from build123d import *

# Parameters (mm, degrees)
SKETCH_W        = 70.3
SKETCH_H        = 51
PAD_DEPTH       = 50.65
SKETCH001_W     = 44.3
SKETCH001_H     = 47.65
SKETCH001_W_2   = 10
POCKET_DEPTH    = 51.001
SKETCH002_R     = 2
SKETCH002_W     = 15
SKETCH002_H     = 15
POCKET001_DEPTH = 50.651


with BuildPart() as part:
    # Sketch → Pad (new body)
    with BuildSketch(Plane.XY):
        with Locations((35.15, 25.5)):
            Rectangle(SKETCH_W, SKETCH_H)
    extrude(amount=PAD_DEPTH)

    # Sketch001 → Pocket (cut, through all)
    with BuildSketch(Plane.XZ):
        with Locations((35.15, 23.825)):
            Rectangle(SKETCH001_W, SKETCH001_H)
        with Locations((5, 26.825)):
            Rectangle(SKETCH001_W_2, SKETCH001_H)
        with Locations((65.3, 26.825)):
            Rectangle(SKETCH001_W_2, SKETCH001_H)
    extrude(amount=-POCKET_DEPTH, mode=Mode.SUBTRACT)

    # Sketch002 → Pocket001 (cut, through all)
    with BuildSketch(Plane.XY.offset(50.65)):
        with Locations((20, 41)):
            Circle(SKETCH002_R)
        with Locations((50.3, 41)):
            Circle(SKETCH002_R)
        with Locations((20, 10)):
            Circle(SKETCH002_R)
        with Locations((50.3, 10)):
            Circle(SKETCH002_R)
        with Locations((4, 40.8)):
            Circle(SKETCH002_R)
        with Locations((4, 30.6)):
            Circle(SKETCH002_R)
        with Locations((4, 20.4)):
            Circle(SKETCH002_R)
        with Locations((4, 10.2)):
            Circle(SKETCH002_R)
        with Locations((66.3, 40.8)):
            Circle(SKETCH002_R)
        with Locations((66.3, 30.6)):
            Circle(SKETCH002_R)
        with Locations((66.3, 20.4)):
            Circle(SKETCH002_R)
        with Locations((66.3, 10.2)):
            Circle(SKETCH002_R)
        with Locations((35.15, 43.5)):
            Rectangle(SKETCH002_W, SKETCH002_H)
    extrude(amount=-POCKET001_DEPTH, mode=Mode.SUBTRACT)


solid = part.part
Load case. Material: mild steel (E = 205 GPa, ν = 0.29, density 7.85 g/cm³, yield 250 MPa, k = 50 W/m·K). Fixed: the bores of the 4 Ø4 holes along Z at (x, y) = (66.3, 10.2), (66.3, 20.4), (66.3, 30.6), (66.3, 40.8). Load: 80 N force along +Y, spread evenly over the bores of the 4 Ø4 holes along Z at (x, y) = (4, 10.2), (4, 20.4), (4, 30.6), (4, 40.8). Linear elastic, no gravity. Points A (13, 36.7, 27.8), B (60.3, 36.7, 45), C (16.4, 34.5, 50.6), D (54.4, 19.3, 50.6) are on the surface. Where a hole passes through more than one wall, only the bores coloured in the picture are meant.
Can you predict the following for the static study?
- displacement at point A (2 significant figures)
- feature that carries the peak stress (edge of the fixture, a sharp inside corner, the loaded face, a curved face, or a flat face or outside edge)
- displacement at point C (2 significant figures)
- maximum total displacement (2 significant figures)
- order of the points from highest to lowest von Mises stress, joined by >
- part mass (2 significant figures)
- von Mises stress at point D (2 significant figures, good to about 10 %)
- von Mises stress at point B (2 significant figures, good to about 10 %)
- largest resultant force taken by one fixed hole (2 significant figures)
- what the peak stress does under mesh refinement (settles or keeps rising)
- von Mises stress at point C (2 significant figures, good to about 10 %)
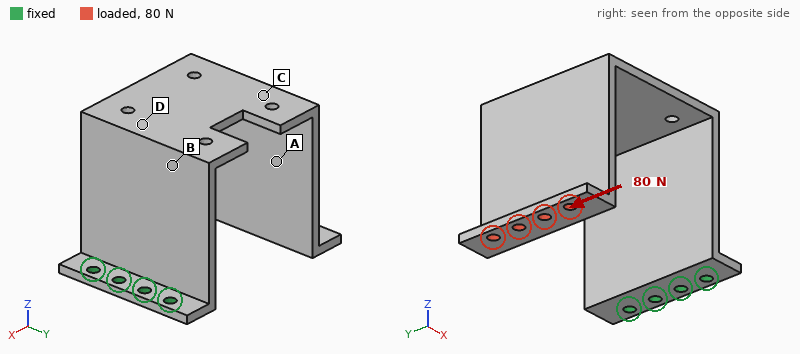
0.36 mm
a sharp inside corner
0.20 mm
0.61 mm
D > B > C > A
190 g
57 MPa
43 MPa
140 N
keeps rising
27 MPa
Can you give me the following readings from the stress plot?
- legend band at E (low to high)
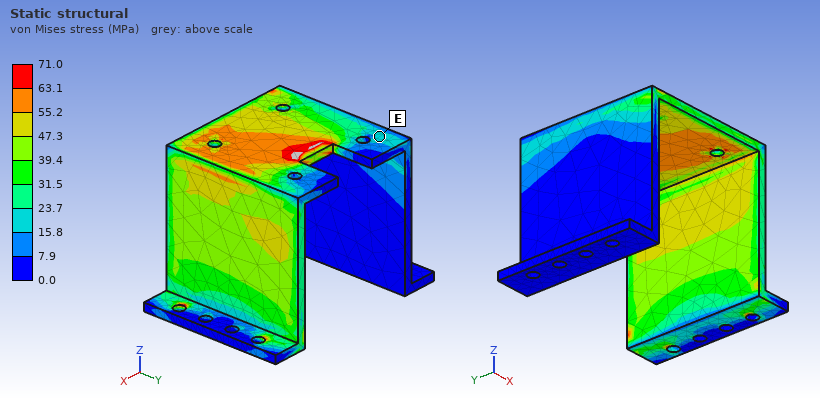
15.8 to 23.7 MPa
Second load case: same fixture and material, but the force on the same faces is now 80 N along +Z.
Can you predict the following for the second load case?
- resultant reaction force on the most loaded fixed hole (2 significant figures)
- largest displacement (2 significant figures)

41 N
1.0 mm
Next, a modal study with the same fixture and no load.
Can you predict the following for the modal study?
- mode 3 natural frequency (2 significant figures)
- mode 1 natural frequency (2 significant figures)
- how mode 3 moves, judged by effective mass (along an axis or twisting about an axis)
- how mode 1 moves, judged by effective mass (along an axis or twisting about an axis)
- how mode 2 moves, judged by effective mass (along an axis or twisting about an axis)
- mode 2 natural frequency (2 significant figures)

340 Hz
180 Hz
along X
along Z
along Y
280 Hz
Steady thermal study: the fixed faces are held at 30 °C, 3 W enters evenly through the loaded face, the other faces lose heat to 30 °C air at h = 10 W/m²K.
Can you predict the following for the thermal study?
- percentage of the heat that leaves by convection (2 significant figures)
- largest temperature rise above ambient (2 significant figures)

73 %
32 K
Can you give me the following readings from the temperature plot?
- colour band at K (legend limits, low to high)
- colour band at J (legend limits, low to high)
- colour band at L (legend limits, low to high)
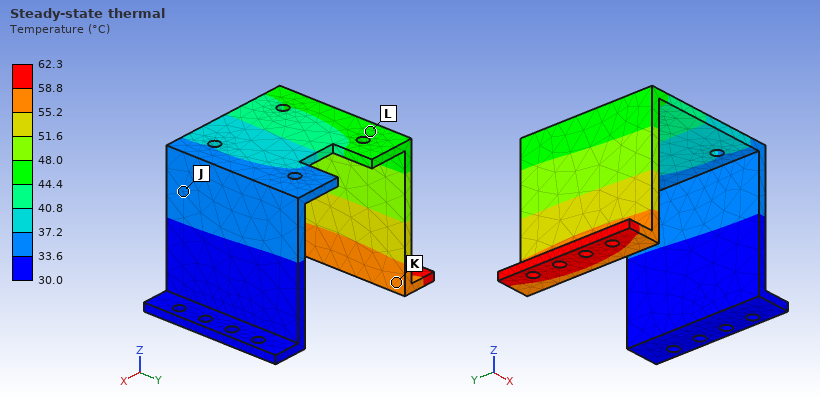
55.2 to 58.8 °C
33.6 to 37.2 °C
44.4 to 48.0 °C
